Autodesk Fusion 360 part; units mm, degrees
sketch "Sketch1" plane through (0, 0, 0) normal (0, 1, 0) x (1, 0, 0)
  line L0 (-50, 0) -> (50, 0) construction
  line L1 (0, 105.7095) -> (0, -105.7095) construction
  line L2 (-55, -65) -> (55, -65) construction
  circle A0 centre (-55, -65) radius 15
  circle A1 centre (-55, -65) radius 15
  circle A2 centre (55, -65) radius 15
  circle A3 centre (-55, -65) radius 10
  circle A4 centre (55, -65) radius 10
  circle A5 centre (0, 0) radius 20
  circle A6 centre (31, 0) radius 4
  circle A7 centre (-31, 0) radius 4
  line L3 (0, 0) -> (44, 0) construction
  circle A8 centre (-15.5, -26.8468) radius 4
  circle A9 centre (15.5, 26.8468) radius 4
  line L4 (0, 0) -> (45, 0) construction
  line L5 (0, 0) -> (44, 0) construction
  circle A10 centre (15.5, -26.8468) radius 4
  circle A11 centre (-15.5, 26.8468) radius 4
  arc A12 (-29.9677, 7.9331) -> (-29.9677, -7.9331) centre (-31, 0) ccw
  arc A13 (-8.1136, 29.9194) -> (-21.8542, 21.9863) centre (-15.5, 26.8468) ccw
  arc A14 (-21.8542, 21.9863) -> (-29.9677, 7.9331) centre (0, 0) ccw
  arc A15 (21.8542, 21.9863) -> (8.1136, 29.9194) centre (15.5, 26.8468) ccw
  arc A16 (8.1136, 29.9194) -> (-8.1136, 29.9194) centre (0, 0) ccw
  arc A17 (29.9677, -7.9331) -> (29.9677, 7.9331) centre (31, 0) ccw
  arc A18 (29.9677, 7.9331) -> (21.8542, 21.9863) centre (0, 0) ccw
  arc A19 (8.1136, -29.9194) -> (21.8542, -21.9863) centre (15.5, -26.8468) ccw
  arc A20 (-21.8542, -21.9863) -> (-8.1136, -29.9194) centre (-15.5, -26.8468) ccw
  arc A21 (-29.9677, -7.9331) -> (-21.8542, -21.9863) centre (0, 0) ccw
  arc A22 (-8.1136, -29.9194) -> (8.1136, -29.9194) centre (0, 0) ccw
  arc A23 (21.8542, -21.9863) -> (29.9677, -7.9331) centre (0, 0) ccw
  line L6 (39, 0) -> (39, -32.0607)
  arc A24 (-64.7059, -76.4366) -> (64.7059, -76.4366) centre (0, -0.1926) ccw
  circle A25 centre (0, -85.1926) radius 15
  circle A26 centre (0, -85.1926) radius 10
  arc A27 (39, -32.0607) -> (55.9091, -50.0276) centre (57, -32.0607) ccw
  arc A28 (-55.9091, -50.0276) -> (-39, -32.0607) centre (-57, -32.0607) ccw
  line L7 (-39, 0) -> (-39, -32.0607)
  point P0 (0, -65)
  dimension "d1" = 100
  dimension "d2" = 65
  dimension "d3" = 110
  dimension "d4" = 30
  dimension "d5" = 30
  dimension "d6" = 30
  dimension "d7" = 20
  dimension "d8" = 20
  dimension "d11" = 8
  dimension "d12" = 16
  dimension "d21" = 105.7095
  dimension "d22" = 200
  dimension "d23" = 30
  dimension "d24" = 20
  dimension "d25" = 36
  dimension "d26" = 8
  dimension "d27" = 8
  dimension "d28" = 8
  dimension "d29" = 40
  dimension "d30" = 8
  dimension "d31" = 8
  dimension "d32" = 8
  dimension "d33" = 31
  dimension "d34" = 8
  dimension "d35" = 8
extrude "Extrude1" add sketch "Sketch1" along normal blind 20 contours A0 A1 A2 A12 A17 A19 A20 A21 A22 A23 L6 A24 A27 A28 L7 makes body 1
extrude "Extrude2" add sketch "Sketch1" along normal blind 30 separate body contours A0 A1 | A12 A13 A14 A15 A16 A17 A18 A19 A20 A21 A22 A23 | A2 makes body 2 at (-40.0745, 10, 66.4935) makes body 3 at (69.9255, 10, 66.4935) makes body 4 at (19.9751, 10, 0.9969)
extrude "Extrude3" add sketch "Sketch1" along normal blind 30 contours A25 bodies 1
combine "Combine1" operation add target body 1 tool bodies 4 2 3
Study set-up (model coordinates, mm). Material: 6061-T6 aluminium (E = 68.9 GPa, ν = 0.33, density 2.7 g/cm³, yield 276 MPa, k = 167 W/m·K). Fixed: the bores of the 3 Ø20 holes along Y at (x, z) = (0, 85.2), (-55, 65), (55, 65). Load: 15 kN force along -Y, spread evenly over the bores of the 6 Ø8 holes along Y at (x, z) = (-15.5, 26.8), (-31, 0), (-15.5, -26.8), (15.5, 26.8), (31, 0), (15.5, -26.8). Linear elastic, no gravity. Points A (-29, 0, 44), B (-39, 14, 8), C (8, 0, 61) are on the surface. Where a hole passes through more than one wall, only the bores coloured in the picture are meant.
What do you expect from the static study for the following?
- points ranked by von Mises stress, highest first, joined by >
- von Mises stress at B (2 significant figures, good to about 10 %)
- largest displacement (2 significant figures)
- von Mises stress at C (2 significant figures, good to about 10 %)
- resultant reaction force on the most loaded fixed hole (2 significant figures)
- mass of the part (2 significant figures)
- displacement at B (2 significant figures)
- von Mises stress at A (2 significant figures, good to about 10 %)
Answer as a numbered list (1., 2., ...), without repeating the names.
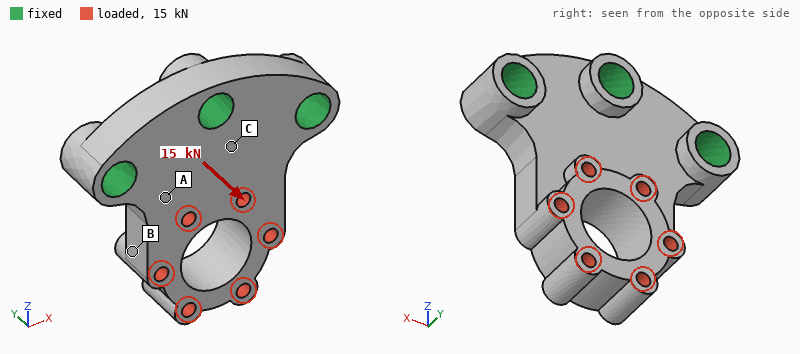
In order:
1. A > C > B
2. 28 MPa
3. 0.85 mm
4. 96 MPa
5. 7.4 kN
6. 580 g
7. 0.34 mm
8. 120 MPa
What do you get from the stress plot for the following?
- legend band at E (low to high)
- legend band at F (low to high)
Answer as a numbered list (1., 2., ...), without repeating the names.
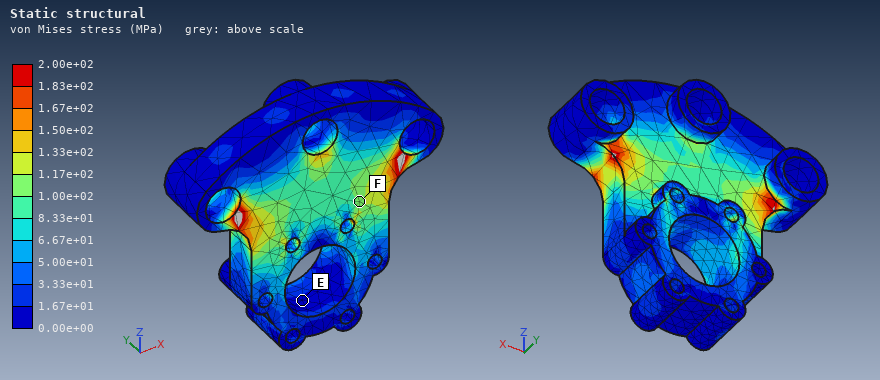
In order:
1. 0.00e+00 to 1.67e+01 MPa
2. 1.00e+02 to 1.17e+02 MPa
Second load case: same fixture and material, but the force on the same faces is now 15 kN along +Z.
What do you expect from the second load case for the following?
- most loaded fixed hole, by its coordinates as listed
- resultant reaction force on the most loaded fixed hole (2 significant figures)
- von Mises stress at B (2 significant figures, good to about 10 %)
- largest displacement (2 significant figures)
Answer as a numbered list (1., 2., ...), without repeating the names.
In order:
1. (0, 85.2)
2. 7.5 kN
3. 9.4 MPa
4. 89 µm
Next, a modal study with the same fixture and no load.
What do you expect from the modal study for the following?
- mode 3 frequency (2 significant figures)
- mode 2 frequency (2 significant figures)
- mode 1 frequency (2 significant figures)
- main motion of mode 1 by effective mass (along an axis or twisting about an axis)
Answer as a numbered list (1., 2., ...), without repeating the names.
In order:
1. 5200 Hz
2. 5100 Hz
3. 1900 Hz
4. along Y
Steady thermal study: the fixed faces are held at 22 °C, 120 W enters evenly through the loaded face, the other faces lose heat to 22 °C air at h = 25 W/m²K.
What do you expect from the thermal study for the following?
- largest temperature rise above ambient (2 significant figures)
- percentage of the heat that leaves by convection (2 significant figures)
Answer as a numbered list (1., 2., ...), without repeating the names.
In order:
1. 38 K
2. 10 %
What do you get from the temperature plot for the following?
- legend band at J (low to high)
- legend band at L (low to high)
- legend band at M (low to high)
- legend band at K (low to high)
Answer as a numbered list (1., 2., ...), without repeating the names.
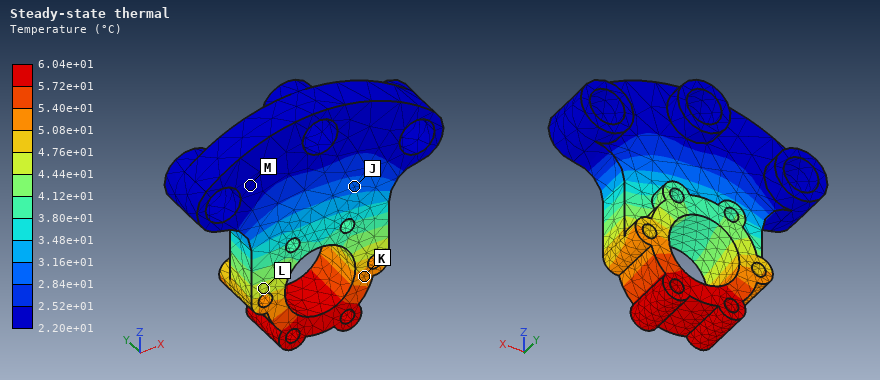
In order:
1. 2.84e+01 to 3.16e+01 °C
2. 4.44e+01 to 4.76e+01 °C
3. 2.20e+01 to 2.52e+01 °C
4. 5.08e+01 to 5.40e+01 °C
